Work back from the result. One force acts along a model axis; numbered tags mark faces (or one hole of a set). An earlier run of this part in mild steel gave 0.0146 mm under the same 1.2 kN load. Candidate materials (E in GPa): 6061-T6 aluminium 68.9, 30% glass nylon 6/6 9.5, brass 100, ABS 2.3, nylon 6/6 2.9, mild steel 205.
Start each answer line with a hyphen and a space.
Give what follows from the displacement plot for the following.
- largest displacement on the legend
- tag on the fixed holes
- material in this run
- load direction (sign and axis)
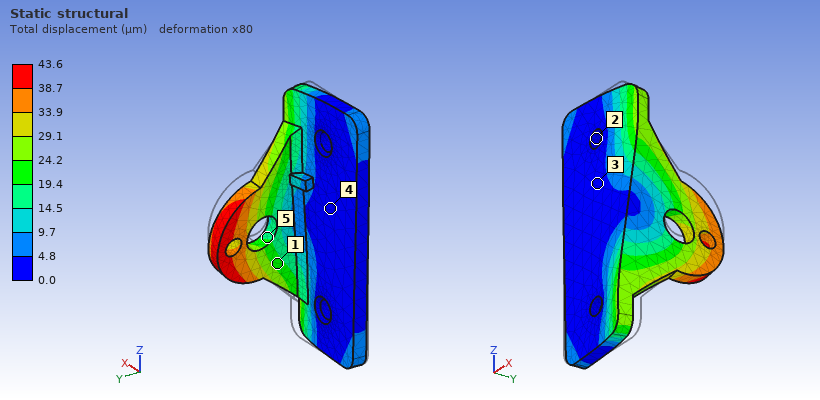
- 43.6 µm
- 2
- 6061-T6 aluminium
- -Z
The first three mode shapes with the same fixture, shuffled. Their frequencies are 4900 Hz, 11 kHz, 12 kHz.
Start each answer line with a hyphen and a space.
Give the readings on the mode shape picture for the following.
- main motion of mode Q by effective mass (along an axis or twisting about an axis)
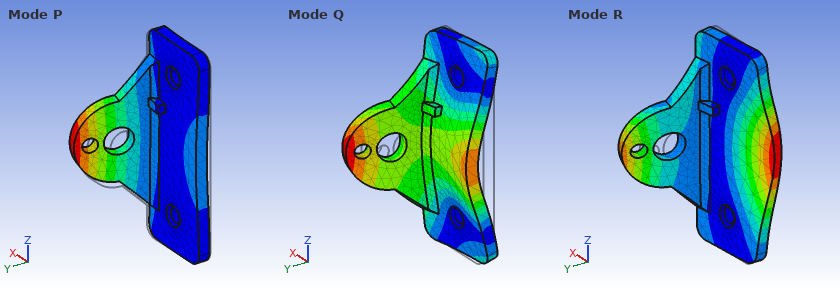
- along Y
